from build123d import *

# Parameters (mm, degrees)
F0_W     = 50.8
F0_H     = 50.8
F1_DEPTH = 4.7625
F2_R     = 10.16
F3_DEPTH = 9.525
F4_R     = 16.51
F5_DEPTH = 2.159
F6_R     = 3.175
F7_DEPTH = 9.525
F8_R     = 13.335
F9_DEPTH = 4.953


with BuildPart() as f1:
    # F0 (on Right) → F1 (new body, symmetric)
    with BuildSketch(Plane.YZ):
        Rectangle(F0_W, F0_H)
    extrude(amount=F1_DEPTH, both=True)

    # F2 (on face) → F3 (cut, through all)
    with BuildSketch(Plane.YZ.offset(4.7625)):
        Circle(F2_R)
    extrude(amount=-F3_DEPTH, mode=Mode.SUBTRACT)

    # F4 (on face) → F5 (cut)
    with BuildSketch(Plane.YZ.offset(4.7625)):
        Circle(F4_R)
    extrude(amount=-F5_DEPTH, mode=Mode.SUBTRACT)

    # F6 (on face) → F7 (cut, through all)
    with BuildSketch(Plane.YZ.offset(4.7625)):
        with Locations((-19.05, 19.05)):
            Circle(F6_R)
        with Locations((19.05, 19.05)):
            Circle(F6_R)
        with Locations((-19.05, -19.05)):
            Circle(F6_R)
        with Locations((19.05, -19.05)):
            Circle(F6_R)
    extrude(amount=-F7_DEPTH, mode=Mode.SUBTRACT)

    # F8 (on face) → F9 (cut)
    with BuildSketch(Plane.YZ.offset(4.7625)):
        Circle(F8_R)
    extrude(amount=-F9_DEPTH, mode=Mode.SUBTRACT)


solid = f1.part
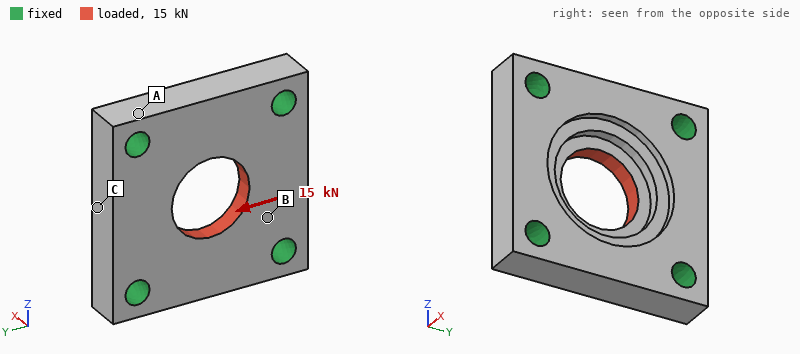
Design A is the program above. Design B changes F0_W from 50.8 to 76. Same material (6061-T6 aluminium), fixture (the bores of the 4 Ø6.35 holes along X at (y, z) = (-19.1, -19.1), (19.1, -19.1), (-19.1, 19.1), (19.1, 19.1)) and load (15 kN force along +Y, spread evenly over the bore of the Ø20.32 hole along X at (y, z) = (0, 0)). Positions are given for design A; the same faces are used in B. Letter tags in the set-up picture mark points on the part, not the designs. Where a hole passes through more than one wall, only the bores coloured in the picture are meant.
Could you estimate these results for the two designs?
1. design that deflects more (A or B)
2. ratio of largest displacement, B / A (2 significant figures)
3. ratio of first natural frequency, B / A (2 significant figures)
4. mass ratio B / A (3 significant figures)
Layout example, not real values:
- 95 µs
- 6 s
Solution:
- A
- 0.80
- 0.60
- 1.66
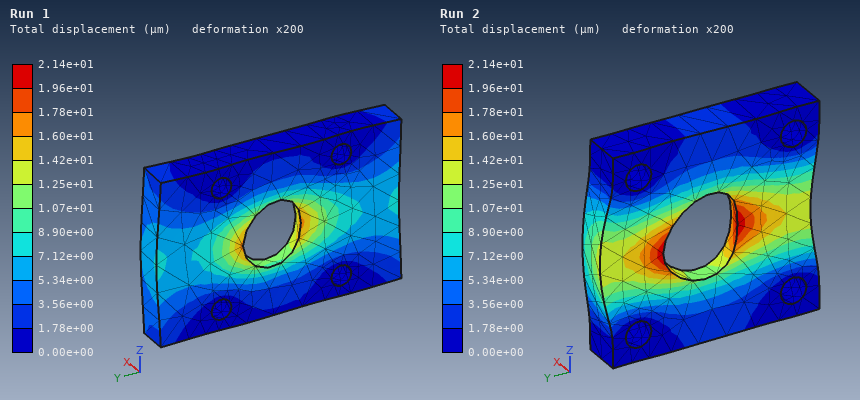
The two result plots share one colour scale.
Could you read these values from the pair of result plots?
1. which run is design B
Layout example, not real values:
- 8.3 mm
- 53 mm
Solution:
- Run 1
